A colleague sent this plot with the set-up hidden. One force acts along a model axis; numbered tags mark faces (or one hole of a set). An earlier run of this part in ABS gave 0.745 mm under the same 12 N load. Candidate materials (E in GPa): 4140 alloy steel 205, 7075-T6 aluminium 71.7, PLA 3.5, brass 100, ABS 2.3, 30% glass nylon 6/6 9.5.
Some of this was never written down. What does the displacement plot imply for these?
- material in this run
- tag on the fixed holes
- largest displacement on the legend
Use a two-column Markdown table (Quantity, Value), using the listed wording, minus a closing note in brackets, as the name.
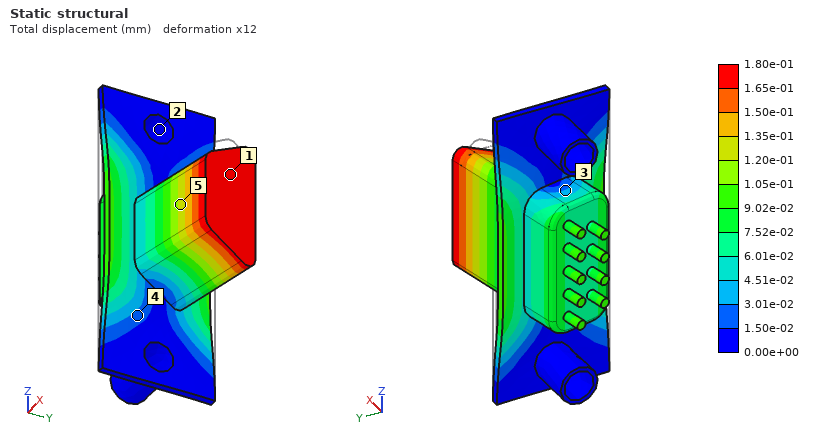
| Quantity | Value |
|---|---|
| material in this run | 30% glass nylon 6/6 |
| tag on the fixed holes | 2 |
| largest displacement on the legend | 1.80e-01 mm |
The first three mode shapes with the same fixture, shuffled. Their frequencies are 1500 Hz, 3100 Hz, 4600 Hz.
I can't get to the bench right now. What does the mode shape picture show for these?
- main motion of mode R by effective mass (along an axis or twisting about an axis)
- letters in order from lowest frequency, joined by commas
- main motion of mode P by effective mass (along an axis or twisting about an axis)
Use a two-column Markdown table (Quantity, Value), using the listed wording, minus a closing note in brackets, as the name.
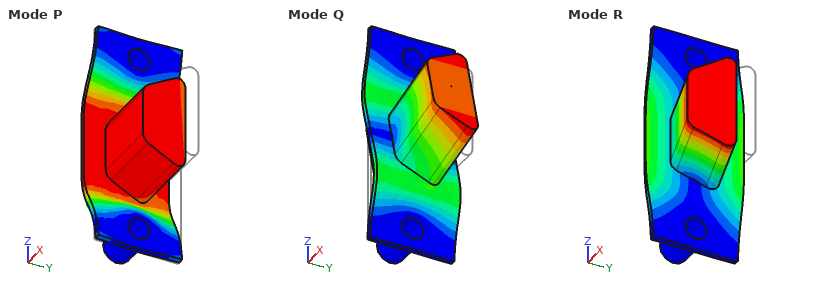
| Quantity | Value |
|---|---|
| main motion of mode R by effective mass | along Y |
| letters in order from lowest frequency, joined by commas | R, P, Q |
| main motion of mode P by effective mass | along X |
